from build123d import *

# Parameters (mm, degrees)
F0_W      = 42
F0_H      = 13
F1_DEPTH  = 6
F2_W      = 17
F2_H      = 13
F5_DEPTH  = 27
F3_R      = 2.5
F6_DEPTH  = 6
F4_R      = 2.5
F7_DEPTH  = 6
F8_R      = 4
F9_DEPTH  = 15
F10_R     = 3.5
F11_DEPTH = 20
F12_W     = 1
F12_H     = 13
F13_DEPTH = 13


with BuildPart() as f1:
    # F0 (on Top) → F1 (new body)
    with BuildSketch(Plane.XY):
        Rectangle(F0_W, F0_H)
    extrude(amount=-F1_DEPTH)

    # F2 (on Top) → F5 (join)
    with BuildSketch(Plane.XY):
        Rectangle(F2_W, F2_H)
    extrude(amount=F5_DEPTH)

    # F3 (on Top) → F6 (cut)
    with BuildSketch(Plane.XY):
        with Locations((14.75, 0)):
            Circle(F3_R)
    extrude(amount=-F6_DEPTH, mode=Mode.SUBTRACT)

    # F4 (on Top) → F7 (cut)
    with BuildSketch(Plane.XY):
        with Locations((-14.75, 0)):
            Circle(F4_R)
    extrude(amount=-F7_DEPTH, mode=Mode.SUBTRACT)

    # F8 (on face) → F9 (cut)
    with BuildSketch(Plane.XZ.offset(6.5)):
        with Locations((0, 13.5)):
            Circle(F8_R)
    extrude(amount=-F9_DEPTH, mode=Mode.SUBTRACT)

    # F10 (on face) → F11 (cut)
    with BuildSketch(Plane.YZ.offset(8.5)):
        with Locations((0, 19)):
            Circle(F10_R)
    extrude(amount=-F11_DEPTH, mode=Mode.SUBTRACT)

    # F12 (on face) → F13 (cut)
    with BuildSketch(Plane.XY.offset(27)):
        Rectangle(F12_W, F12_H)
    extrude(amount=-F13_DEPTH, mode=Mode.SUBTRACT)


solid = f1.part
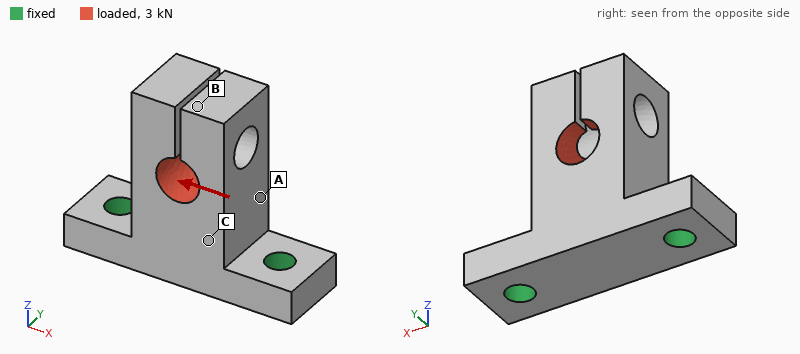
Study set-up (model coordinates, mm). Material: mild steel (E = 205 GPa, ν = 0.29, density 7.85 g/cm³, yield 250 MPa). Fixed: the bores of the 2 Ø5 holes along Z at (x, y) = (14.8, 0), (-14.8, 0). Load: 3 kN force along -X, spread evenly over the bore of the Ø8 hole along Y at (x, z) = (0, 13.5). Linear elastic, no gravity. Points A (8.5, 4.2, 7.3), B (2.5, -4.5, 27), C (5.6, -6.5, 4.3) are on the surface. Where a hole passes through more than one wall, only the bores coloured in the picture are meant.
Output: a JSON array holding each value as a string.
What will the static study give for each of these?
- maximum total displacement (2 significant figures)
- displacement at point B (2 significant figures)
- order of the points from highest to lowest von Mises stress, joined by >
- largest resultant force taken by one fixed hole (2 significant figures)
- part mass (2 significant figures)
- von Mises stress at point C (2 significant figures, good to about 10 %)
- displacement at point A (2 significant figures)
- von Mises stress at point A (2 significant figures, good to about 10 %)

["33 µm", "33 µm", "A > C > B", "2.6 kN", "60 g", "28 MPa", "8.7 µm", "49 MPa"]
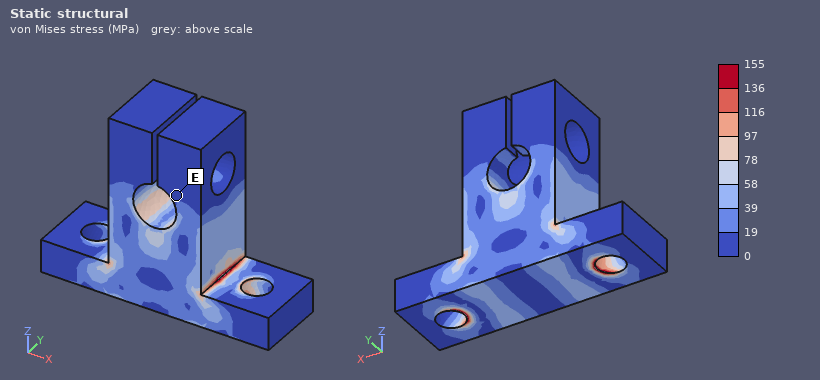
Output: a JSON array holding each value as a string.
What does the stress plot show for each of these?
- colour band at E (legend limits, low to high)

["0 to 19 MPa"]
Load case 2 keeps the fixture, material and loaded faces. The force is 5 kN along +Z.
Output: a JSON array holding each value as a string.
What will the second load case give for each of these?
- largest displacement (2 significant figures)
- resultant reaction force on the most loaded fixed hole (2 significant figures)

["26 µm", "2.7 kN"]
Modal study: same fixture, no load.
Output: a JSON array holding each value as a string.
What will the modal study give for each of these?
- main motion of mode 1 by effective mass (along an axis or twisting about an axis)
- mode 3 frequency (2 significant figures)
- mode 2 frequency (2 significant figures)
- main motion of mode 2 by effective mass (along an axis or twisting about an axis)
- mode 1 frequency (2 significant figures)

["along Y", "8300 Hz", "7400 Hz", "along X", "5400 Hz"]
